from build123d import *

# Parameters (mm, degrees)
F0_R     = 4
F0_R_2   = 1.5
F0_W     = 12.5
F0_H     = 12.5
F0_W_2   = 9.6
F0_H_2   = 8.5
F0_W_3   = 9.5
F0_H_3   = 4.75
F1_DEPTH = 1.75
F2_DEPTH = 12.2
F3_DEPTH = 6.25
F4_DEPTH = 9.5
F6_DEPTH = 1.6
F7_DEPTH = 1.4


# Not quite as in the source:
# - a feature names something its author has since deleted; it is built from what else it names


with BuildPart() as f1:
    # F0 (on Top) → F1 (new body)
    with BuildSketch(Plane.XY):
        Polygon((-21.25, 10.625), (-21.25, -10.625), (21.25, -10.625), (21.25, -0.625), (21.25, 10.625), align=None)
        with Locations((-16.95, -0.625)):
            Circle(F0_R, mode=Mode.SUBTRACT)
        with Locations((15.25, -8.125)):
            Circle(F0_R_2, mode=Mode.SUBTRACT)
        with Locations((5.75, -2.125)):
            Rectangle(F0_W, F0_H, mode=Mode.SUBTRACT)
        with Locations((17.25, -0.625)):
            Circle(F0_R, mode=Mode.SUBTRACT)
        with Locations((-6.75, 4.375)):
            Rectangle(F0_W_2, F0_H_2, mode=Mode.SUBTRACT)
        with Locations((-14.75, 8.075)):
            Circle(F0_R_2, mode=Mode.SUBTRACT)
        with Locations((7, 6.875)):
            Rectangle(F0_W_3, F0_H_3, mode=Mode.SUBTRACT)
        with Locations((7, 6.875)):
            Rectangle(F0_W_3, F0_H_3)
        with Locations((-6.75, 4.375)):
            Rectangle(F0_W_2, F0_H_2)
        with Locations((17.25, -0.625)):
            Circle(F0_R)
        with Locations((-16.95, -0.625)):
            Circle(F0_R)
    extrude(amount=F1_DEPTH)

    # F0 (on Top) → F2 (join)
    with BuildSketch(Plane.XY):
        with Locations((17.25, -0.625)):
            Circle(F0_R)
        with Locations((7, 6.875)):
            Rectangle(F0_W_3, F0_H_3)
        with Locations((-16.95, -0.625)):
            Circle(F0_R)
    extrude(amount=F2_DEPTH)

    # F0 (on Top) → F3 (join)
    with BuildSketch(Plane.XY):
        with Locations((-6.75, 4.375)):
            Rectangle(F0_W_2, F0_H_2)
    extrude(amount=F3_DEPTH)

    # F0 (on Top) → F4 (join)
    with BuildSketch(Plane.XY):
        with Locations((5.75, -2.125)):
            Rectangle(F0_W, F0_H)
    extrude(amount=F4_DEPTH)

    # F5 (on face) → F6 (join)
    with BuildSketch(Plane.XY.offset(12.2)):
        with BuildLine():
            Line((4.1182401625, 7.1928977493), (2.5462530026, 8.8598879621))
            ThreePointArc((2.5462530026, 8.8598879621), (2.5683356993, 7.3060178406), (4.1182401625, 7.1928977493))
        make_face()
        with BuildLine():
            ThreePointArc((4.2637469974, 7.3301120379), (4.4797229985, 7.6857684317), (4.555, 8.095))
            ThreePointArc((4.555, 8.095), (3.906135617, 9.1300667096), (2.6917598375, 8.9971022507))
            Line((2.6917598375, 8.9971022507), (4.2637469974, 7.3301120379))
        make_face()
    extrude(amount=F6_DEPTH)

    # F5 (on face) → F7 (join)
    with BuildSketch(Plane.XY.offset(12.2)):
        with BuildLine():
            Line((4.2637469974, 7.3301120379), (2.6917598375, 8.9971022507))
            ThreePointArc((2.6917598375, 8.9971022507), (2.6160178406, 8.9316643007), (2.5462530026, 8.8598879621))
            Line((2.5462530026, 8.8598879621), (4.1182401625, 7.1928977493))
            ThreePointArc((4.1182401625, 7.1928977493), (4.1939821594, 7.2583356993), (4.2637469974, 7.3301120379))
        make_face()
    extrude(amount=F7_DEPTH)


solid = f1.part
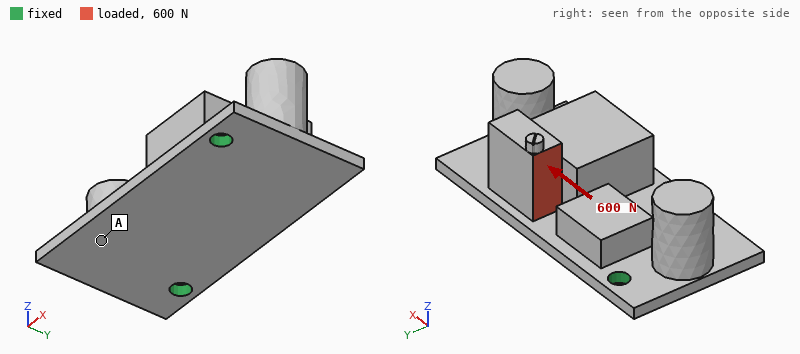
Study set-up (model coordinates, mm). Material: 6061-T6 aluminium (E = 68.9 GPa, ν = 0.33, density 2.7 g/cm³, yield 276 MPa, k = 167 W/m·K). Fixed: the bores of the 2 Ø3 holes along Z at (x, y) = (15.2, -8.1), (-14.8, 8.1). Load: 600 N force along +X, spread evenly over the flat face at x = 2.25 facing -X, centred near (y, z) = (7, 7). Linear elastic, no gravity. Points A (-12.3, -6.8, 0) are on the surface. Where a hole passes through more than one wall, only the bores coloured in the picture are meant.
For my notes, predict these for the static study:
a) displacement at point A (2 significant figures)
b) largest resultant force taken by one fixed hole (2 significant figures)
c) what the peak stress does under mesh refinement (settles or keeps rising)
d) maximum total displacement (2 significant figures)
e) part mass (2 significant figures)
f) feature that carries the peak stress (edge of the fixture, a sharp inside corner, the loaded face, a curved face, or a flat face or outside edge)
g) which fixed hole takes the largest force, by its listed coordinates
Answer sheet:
0.066 mm
370 N
keeps rising
0.14 mm
13 g
edge of the fixture
(-14.8, 8.1)
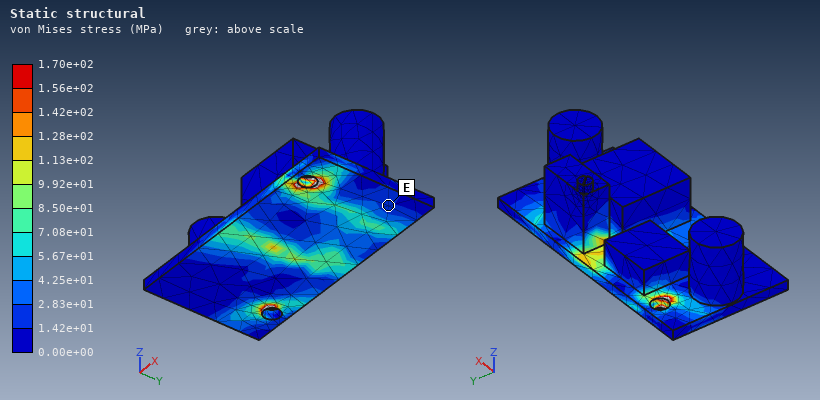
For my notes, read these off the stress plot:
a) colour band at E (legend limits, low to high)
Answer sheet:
1.42e+01 to 2.83e+01 MPa
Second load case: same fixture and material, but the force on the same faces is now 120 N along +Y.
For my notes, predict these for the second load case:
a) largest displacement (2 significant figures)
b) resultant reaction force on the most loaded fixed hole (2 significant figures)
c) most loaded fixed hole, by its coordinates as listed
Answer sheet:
66 µm
69 N
(15.2, -8.1)
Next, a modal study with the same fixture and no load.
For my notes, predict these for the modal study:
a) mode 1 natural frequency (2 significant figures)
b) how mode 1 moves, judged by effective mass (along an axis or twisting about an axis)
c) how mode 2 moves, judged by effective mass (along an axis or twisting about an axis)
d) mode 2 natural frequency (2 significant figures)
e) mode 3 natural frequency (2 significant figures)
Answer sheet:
3200 Hz
along Y
along Z
4700 Hz
5500 Hz
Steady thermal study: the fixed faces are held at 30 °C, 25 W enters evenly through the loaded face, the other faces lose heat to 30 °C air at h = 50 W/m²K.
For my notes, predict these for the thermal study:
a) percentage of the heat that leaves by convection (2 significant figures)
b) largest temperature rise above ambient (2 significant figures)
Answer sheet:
13 %
64 K
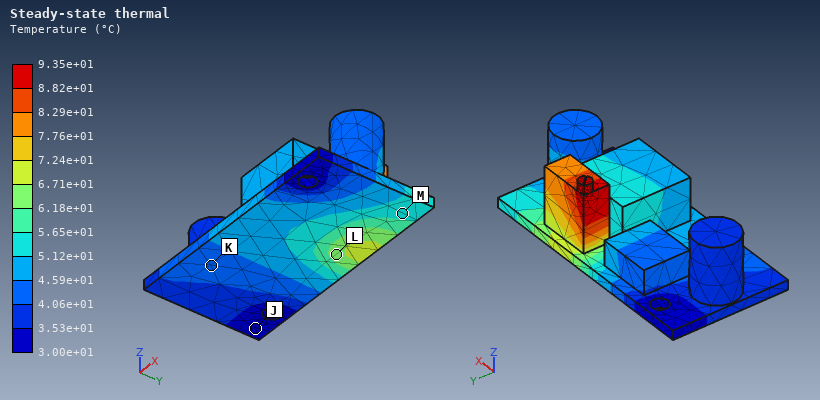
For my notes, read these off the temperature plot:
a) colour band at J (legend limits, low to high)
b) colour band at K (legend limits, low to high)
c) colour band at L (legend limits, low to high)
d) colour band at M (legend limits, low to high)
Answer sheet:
3.00e+01 to 3.53e+01 °C
4.06e+01 to 4.59e+01 °C
6.18e+01 to 6.71e+01 °C
5.12e+01 to 5.65e+01 °C
